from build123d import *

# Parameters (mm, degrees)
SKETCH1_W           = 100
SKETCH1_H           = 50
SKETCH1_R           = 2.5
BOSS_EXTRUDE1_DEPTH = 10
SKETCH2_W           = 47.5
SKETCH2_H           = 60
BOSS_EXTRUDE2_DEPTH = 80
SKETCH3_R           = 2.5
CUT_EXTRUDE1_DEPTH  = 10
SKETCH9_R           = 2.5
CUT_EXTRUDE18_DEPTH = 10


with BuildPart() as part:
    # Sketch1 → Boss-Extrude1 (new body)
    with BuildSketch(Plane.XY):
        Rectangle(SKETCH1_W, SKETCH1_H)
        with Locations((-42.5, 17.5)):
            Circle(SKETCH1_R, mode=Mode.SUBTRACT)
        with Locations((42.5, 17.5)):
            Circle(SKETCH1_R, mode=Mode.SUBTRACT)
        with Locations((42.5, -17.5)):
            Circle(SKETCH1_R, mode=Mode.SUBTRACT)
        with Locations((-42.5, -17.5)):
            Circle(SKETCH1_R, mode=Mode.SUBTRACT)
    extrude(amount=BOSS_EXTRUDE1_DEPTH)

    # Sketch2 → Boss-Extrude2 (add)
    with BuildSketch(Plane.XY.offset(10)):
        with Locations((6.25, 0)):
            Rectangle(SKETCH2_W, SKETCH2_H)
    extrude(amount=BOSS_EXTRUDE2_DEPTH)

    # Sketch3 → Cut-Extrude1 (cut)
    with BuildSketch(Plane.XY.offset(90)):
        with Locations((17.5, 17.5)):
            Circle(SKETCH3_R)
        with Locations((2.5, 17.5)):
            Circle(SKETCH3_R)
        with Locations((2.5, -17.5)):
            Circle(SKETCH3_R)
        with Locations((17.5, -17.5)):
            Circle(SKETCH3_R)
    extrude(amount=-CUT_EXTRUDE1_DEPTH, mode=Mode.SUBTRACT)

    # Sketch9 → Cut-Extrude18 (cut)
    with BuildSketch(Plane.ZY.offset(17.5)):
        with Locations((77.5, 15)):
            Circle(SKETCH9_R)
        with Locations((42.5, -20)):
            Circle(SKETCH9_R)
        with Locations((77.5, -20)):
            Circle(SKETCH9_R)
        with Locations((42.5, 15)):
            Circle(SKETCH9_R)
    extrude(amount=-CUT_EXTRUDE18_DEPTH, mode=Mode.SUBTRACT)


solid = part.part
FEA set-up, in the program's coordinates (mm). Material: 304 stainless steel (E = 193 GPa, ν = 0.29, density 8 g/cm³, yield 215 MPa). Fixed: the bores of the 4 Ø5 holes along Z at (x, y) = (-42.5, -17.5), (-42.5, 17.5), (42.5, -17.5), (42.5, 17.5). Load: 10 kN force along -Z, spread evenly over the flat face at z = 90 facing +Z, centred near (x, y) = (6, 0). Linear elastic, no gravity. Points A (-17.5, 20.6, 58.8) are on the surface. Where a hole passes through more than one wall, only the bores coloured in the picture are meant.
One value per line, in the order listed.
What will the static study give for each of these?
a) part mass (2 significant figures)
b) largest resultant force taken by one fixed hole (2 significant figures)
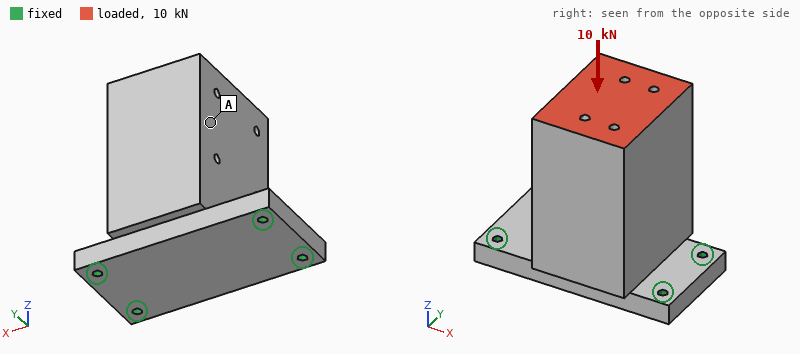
2.2 kg
3.0 kN
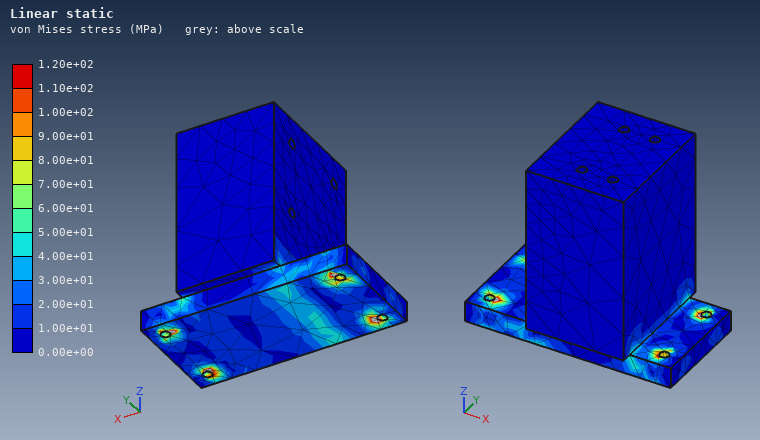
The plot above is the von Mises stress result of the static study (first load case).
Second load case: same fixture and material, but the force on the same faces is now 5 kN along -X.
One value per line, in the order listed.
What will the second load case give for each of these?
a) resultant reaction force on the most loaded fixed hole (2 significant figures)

3.4 kN
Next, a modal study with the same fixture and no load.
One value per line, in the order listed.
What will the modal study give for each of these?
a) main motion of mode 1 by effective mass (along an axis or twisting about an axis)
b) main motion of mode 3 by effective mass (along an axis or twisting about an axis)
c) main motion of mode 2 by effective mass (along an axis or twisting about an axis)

along Y
along Z
along X
